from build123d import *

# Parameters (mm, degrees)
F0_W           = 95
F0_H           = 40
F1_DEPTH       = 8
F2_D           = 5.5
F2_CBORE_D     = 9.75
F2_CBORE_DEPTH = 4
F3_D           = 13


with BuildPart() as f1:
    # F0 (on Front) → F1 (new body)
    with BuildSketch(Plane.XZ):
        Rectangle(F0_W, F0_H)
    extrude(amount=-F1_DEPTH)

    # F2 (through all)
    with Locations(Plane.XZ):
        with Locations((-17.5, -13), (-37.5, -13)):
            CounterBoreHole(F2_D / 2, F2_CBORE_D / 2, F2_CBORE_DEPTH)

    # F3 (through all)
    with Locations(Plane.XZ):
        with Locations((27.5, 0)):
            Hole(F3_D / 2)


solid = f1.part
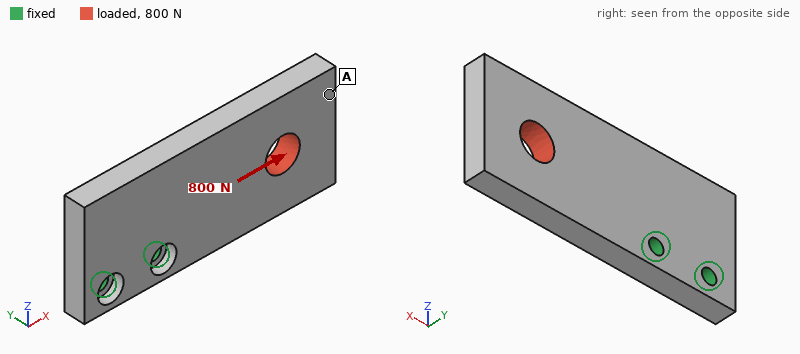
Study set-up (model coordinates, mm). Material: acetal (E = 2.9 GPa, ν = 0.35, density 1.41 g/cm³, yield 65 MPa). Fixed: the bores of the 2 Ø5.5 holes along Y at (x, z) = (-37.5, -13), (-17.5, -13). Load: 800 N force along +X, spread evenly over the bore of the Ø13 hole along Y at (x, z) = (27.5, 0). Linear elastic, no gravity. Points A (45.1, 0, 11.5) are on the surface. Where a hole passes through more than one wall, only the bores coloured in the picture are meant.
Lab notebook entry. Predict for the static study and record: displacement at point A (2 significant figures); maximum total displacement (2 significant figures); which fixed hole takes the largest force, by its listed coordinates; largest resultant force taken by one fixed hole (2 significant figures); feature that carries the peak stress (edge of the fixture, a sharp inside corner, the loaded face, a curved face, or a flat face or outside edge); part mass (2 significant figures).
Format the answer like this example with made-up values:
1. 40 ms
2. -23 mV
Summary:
1. 0.26 mm
2. 0.27 mm
3. (-17.5, -13)
4. 660 N
5. edge of the fixture
6. 40 g
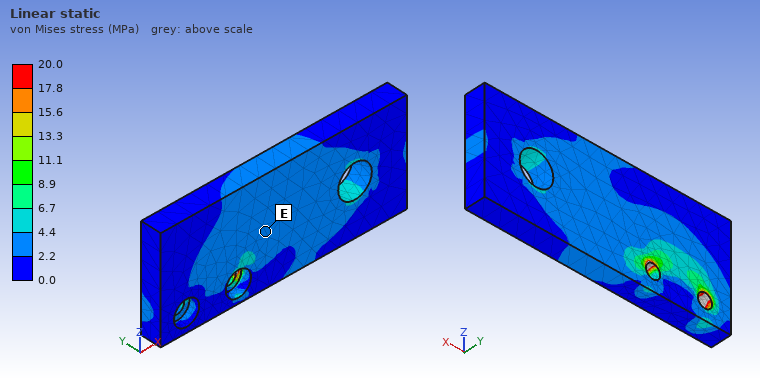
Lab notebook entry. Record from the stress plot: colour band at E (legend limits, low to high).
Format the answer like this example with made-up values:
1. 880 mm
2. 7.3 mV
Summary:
1. 2.2 to 4.4 MPa
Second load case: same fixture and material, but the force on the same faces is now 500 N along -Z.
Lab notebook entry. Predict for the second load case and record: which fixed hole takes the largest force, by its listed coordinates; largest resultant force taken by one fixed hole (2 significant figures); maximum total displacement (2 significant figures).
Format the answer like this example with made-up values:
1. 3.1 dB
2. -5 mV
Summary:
1. (-17.5, -13)
2. 1.4 kN
3. 1.1 mm
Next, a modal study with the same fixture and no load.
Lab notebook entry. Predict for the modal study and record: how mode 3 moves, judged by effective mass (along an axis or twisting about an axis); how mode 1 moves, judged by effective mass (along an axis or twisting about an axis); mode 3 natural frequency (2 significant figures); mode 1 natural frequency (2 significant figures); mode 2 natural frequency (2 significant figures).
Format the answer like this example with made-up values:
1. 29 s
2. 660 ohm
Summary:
1. along Z
2. along Y
3. 990 Hz
4. 340 Hz
5. 800 Hz
